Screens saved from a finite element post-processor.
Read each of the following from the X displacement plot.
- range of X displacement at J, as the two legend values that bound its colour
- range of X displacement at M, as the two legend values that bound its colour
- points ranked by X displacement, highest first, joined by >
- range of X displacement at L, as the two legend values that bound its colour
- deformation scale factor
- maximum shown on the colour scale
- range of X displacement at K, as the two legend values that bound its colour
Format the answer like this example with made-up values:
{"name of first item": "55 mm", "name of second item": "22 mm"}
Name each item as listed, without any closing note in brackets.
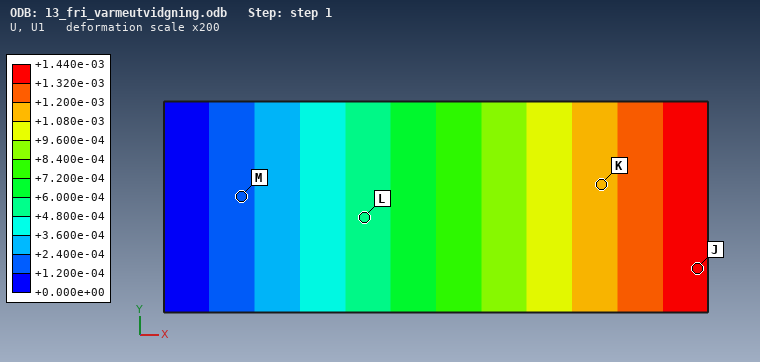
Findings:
{"range of X displacement at J, as the two legend values that bound its colour": "+1.320e-03 to +1.440e-03", "range of X displacement at M, as the two legend values that bound its colour": "+1.200e-04 to +2.400e-04", "points ranked by X displacement, highest first, joined by >": "J > K > L > M", "range of X displacement at L, as the two legend values that bound its colour": "+4.800e-04 to +6.000e-04", "deformation scale factor": "200", "maximum shown on the colour scale": "+1.440e-03", "range of X displacement at K, as the two legend values that bound its colour": "+1.080e-03 to +1.200e-03"}
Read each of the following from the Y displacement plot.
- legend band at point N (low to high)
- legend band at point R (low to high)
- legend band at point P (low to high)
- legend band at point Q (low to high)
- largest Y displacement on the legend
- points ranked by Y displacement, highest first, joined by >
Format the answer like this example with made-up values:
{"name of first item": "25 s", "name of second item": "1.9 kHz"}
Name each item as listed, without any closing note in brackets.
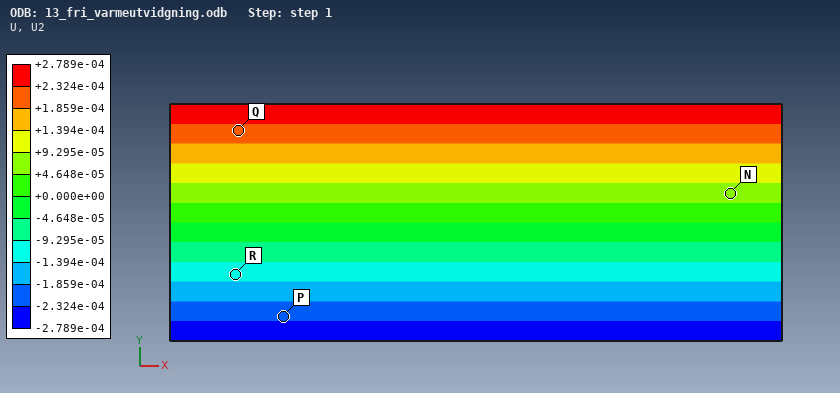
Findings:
{"legend band at point N": "+4.648e-05 to +9.295e-05", "legend band at point R": "-1.394e-04 to -9.295e-05", "legend band at point P": "-2.324e-04 to -1.859e-04", "legend band at point Q": "+1.859e-04 to +2.324e-04", "largest Y displacement on the legend": "+2.789e-04", "points ranked by Y displacement, highest first, joined by >": "Q > N > R > P"}
